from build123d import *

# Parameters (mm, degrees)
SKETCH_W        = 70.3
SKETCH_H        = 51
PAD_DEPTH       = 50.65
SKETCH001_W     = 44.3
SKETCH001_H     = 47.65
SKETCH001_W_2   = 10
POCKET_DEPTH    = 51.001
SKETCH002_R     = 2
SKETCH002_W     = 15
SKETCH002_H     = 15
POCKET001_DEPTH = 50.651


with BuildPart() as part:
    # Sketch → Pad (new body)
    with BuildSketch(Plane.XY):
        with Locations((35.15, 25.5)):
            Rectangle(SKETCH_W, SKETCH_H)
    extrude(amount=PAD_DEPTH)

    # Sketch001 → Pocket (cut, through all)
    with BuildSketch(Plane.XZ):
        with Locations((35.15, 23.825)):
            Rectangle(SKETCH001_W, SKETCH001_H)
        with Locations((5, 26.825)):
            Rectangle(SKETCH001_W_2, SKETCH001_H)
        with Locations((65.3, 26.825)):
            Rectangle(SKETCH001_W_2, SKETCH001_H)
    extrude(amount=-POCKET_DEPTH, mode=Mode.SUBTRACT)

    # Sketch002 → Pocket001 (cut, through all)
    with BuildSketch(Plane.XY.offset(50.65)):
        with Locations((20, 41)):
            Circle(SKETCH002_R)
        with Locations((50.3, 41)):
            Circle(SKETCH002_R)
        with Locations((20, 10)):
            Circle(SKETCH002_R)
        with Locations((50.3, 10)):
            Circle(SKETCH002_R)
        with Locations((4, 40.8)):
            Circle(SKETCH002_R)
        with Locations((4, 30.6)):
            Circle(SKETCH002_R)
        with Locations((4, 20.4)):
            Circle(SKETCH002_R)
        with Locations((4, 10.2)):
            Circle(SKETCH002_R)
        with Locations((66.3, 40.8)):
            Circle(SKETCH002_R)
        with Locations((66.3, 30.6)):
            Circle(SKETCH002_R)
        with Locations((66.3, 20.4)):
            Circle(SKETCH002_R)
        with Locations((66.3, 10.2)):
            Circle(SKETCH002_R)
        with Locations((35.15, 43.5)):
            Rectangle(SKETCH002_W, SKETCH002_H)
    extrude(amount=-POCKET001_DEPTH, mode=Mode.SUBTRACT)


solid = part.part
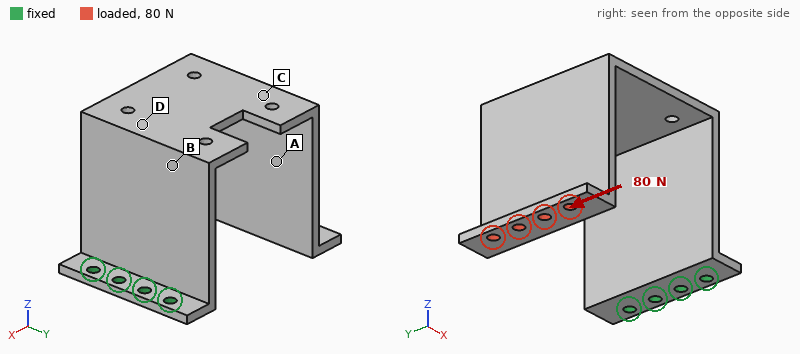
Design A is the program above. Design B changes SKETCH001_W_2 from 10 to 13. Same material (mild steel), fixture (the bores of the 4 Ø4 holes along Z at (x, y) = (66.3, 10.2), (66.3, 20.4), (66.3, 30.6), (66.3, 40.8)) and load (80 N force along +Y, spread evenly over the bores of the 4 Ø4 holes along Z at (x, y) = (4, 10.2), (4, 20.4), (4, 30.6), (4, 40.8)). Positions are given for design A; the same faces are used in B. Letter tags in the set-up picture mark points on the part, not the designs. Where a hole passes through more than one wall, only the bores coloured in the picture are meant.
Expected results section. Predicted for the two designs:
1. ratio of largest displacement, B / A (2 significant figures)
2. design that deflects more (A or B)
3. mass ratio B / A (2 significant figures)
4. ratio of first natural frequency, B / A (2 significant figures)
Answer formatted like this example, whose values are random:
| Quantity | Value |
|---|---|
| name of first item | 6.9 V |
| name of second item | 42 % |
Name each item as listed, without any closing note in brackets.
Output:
| Quantity | Value |
|---|---|
| ratio of largest displacement, B / A | 3.3 |
| design that deflects more | B |
| mass ratio B / A | 0.70 |
| ratio of first natural frequency, B / A | 0.53 |
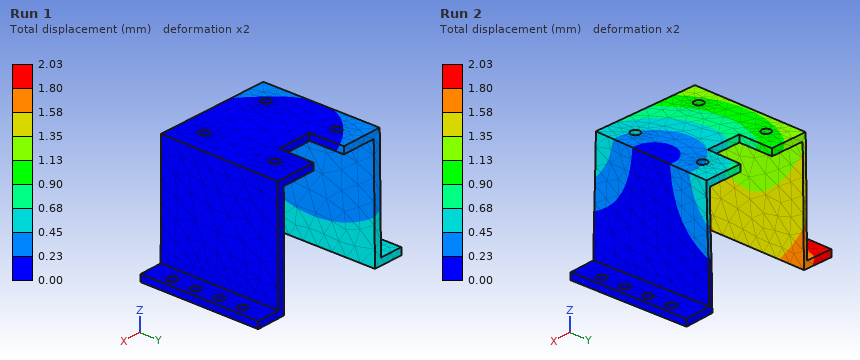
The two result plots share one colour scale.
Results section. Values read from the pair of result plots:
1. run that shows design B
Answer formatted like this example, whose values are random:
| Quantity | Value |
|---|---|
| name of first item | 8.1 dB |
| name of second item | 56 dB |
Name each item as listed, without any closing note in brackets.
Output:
| Quantity | Value |
|---|---|
| run that shows design B | Run 2 |
